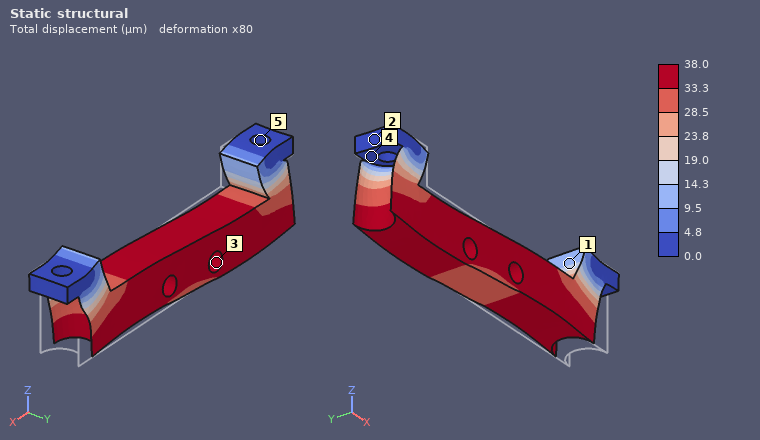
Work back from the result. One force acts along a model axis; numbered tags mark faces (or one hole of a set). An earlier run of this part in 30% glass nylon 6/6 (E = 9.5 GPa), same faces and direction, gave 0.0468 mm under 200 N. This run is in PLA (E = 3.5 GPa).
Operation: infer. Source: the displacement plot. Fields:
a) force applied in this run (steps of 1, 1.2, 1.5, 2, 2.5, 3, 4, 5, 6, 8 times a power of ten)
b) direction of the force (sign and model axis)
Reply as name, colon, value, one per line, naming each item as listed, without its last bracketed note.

force applied in this run: 60 N
direction of the force: -X
